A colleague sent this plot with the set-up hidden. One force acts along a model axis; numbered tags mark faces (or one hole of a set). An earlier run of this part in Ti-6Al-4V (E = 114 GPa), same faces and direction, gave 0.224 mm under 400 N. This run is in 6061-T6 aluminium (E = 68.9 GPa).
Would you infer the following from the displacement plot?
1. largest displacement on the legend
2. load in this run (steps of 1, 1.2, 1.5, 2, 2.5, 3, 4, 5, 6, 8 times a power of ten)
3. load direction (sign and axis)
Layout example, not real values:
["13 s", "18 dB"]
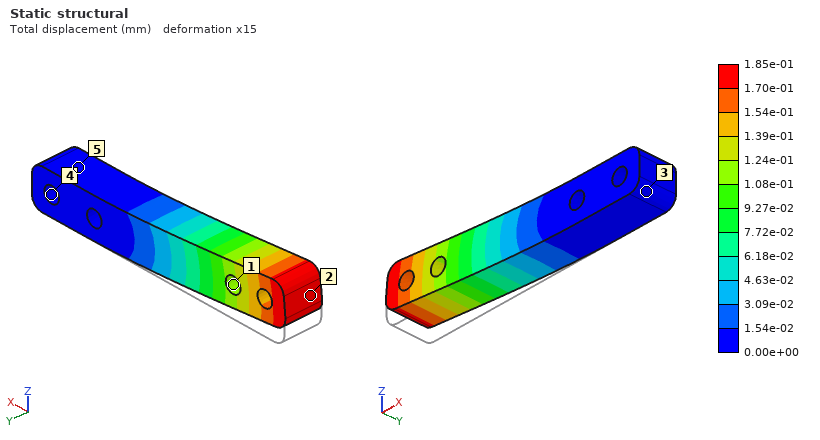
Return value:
["1.85e-01 mm", "200 N", "+Z"]
